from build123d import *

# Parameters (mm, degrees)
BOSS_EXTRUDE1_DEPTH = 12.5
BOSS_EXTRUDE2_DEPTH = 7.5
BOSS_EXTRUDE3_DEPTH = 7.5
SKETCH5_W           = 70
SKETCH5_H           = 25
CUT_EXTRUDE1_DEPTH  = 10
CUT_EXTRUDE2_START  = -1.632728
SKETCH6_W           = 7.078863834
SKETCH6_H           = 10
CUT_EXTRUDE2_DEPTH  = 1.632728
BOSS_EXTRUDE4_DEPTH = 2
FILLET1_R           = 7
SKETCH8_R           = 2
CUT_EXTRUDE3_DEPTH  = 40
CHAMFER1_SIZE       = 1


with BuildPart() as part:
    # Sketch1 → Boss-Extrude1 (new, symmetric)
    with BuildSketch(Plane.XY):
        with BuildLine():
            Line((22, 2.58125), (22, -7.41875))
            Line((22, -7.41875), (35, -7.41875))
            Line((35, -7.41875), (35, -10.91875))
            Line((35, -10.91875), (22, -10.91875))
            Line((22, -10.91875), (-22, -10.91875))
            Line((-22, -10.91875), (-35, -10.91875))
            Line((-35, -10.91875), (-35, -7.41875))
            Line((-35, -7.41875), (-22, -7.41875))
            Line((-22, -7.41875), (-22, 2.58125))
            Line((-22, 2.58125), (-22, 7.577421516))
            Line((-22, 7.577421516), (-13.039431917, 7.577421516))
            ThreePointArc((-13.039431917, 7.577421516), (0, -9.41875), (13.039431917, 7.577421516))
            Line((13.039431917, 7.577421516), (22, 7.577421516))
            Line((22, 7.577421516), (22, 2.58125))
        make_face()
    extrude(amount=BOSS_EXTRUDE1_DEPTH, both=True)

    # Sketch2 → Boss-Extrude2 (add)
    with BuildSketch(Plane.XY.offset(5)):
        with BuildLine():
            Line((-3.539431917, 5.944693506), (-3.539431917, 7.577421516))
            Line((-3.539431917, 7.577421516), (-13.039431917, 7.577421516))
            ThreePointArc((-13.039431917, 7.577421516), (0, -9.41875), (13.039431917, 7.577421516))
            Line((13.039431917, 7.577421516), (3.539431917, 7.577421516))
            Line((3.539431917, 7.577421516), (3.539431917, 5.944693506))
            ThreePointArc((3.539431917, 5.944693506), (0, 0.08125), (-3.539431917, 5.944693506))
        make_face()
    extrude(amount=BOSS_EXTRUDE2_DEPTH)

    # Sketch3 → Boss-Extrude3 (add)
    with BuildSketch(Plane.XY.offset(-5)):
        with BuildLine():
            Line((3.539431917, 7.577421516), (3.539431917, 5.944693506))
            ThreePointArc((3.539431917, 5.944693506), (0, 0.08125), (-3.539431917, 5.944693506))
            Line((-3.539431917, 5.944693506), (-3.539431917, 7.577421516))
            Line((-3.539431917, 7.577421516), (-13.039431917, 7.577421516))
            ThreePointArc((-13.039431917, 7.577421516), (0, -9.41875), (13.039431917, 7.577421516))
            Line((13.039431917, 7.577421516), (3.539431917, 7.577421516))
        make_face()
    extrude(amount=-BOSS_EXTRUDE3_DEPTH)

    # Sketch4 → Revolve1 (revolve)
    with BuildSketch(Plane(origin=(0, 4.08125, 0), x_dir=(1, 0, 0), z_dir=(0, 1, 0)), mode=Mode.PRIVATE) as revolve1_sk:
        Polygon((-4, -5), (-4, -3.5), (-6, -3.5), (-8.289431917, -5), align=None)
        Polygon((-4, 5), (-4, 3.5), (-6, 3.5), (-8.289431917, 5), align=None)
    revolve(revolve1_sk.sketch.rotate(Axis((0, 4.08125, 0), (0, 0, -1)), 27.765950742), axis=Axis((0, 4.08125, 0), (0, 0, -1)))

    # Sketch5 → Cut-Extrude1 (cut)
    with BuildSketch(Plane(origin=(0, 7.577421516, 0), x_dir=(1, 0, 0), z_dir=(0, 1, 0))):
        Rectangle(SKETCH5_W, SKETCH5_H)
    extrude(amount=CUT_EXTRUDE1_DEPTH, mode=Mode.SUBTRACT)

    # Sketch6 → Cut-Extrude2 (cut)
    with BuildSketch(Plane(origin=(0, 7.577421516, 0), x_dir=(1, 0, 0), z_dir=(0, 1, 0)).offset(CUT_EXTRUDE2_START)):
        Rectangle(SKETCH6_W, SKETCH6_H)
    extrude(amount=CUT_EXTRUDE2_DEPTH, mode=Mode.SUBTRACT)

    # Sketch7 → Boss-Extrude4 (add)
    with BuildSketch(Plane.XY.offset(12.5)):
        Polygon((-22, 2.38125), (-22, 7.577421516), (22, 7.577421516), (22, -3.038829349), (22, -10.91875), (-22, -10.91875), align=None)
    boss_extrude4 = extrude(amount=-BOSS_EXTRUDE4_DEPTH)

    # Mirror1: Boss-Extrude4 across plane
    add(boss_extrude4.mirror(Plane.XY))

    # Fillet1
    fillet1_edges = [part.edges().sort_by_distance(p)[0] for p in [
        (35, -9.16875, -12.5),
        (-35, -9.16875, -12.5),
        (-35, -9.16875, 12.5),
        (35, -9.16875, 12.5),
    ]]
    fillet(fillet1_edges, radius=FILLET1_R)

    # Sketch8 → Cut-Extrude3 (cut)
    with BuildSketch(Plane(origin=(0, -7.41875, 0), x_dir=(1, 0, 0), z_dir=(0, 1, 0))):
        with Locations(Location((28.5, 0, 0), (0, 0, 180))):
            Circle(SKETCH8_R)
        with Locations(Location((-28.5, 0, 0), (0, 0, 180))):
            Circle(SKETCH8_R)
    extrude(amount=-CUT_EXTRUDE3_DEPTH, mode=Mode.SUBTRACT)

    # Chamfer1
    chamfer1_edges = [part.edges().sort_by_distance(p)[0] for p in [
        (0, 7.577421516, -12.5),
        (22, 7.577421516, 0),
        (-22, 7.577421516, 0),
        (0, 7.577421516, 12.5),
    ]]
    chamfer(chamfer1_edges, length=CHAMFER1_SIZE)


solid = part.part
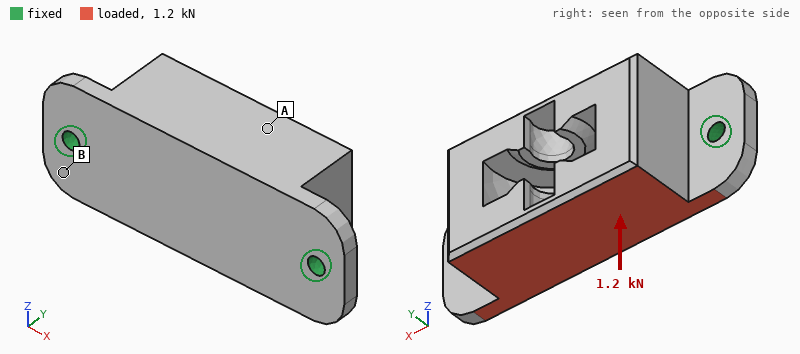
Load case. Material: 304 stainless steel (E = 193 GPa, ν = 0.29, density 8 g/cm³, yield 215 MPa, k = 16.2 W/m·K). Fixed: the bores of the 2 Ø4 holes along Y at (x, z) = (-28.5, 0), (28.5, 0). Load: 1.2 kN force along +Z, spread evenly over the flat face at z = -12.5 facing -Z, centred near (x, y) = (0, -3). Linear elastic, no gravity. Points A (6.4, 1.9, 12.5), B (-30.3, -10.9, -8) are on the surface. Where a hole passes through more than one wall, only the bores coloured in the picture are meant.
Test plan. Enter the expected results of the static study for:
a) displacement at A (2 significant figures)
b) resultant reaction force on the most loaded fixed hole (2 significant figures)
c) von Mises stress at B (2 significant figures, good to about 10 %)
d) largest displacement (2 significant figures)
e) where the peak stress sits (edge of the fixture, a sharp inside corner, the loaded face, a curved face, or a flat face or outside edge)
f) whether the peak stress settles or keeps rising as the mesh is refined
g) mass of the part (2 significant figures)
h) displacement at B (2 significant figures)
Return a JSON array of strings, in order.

["18 µm", "600 N", "25 MPa", "24 µm", "edge of the fixture", "keeps rising", "150 g", "4.0 µm"]
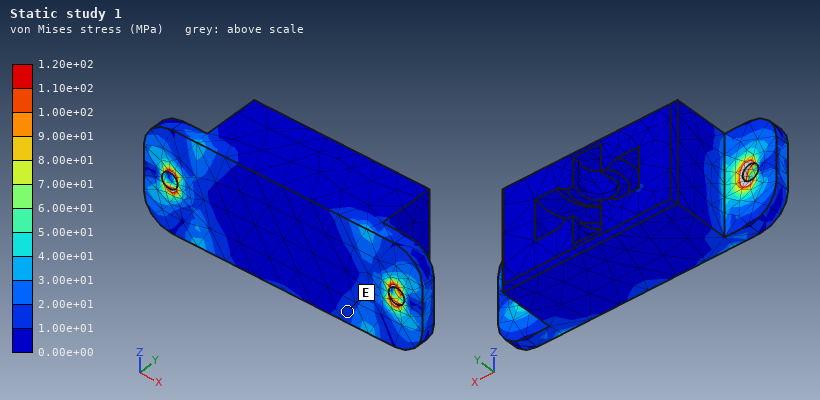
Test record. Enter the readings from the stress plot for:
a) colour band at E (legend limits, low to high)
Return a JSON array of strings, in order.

["1.00e+01 to 2.00e+01 MPa"]
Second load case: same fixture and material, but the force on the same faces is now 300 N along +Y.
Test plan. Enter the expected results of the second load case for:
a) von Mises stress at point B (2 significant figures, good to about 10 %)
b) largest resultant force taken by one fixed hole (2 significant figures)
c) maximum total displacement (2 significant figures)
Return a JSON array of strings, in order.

["14 MPa", "180 N", "11 µm"]
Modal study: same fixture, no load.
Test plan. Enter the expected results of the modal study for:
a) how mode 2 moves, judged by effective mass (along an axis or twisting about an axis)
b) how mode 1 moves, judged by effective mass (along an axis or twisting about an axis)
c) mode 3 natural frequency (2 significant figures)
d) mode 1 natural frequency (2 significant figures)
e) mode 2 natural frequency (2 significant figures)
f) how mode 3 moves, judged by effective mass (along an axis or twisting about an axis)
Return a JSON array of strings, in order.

["along Y", "along Z", "12 kHz", "3300 Hz", "7300 Hz", "along X"]
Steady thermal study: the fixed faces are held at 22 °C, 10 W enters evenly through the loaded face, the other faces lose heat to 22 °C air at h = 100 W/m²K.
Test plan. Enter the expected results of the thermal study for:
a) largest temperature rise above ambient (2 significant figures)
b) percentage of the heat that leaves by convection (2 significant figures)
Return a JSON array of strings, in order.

["27 K", "72 %"]
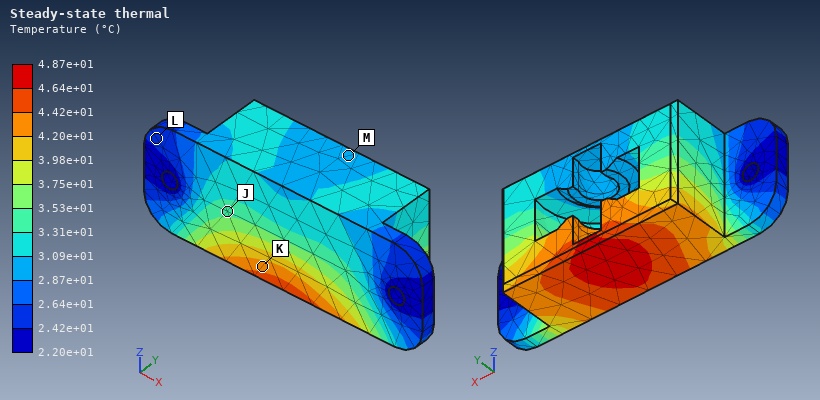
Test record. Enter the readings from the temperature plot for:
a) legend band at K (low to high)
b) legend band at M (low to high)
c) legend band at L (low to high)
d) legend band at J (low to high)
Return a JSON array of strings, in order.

["4.20e+01 to 4.42e+01 °C", "2.87e+01 to 3.09e+01 °C", "2.42e+01 to 2.64e+01 °C", "3.31e+01 to 3.53e+01 °C"]
